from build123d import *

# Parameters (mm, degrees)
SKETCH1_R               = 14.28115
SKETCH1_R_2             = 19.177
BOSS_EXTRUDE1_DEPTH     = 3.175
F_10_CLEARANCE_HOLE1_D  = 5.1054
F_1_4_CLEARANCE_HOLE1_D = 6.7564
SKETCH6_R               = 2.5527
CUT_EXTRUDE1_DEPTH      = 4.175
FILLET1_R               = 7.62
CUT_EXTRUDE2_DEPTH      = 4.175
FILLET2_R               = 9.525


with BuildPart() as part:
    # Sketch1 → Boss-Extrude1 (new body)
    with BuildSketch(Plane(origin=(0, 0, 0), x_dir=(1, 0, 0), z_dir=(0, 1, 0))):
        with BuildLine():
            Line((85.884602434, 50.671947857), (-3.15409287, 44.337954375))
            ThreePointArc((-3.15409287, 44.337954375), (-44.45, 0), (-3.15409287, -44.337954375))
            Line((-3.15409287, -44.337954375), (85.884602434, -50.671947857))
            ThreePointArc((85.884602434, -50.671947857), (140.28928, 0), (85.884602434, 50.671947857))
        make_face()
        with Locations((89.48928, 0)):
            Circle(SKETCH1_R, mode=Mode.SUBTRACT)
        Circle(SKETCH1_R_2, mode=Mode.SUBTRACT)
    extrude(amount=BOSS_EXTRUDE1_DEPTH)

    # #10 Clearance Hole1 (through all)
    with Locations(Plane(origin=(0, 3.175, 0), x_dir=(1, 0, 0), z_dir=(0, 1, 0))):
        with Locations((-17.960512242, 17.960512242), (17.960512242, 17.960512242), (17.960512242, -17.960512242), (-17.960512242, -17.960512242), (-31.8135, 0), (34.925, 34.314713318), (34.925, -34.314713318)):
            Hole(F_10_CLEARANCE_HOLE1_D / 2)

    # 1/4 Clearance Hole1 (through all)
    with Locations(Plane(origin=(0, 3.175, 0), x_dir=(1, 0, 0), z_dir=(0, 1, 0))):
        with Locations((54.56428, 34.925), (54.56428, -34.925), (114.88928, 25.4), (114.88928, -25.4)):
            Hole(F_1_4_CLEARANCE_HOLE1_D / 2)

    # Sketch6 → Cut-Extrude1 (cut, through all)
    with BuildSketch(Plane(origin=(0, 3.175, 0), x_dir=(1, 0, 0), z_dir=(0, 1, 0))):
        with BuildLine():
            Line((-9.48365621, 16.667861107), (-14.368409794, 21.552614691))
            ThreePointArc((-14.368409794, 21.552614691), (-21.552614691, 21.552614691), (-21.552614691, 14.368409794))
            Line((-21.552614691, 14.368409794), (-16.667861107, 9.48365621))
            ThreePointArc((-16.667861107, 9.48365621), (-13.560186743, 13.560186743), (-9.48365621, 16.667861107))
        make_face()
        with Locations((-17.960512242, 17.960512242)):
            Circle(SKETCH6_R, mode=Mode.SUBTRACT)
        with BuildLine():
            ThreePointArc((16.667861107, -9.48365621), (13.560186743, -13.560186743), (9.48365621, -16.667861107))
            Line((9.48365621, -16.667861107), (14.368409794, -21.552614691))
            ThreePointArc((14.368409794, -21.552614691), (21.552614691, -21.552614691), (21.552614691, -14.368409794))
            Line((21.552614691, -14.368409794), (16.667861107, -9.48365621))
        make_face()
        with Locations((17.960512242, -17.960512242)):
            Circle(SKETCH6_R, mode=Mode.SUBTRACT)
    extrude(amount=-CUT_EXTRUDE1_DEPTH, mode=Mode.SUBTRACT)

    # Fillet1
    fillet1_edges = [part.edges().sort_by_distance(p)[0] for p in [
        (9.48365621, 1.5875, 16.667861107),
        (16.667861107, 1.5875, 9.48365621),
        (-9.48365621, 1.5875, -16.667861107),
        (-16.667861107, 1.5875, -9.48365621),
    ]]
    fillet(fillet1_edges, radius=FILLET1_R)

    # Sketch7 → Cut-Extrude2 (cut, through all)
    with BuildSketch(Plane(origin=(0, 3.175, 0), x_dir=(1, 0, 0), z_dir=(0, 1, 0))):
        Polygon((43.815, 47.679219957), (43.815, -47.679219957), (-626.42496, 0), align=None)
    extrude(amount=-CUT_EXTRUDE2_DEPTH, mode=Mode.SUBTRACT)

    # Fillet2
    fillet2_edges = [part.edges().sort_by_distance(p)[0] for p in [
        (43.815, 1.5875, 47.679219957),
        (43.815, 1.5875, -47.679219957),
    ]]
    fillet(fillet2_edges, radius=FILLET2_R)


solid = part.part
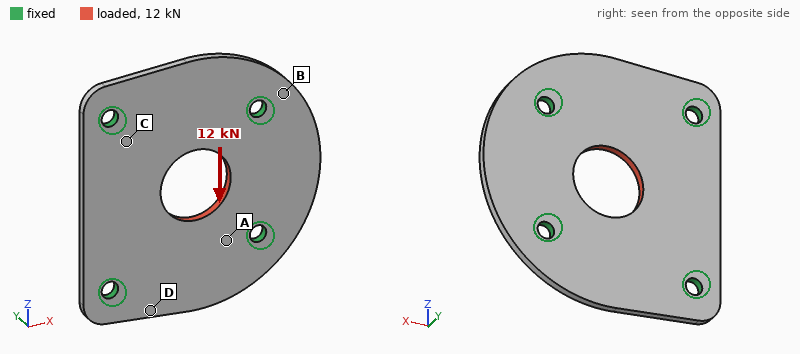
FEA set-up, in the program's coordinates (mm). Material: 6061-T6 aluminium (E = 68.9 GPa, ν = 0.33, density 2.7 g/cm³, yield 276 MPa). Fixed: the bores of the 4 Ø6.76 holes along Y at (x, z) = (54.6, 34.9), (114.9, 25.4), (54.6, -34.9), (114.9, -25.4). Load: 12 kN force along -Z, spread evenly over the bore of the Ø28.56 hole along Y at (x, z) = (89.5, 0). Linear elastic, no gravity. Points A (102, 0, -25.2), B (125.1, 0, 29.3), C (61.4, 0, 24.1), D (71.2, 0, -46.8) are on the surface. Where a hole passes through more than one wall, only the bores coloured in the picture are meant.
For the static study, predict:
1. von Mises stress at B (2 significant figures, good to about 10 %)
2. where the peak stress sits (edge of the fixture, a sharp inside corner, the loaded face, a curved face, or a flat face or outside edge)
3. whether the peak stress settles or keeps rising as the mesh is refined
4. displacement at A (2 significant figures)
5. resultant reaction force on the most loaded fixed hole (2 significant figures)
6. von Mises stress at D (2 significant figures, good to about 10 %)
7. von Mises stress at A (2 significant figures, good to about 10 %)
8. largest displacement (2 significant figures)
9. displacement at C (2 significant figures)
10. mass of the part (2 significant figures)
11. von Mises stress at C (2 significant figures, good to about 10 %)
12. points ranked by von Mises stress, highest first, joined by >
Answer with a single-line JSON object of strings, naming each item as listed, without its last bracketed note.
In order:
{"von Mises stress at B": "9.3 MPa", "where the peak stress sits": "edge of the fixture", "whether the peak stress settles or keeps rising as the mesh is refined": "keeps rising", "displacement at A": "14 µm", "resultant reaction force on the most loaded fixed hole": "3.4 kN", "von Mises stress at D": "19 MPa", "von Mises stress at A": "33 MPa", "largest displacement": "27 µm", "displacement at C": "8.2 µm", "mass of the part": "66 g", "von Mises stress at C": "43 MPa", "points ranked by von Mises stress, highest first, joined by >": "C > A > D > B"}
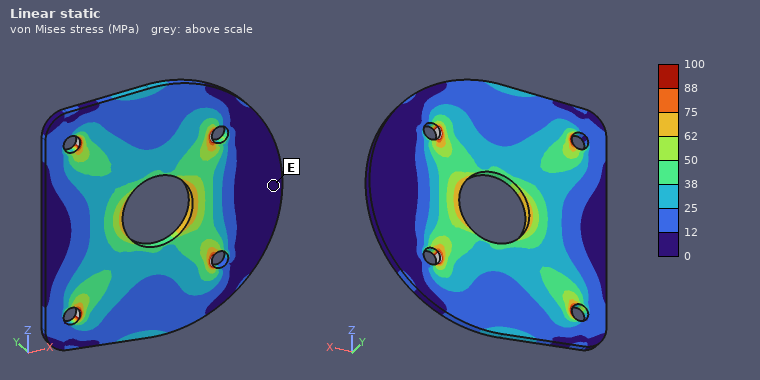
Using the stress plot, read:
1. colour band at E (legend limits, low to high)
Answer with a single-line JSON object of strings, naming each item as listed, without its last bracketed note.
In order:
{"colour band at E": "0 to 12 MPa"}
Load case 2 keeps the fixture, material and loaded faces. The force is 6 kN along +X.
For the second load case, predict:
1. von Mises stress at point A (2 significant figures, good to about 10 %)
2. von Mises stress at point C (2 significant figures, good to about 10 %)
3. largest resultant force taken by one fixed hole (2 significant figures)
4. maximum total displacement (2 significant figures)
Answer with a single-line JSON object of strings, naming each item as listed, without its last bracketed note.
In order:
{"von Mises stress at point A": "22 MPa", "von Mises stress at point C": "20 MPa", "largest resultant force taken by one fixed hole": "1.9 kN", "maximum total displacement": "16 µm"}
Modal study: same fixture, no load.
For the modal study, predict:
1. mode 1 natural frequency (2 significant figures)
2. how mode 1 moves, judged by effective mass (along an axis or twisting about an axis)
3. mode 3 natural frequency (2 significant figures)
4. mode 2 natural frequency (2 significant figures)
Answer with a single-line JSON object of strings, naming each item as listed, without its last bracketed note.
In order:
{"mode 1 natural frequency": "3500 Hz", "how mode 1 moves, judged by effective mass": "along Y", "mode 3 natural frequency": "4000 Hz", "mode 2 natural frequency": "3900 Hz"}
